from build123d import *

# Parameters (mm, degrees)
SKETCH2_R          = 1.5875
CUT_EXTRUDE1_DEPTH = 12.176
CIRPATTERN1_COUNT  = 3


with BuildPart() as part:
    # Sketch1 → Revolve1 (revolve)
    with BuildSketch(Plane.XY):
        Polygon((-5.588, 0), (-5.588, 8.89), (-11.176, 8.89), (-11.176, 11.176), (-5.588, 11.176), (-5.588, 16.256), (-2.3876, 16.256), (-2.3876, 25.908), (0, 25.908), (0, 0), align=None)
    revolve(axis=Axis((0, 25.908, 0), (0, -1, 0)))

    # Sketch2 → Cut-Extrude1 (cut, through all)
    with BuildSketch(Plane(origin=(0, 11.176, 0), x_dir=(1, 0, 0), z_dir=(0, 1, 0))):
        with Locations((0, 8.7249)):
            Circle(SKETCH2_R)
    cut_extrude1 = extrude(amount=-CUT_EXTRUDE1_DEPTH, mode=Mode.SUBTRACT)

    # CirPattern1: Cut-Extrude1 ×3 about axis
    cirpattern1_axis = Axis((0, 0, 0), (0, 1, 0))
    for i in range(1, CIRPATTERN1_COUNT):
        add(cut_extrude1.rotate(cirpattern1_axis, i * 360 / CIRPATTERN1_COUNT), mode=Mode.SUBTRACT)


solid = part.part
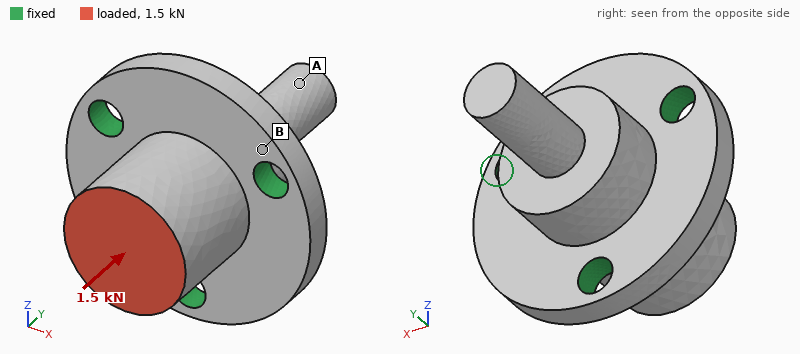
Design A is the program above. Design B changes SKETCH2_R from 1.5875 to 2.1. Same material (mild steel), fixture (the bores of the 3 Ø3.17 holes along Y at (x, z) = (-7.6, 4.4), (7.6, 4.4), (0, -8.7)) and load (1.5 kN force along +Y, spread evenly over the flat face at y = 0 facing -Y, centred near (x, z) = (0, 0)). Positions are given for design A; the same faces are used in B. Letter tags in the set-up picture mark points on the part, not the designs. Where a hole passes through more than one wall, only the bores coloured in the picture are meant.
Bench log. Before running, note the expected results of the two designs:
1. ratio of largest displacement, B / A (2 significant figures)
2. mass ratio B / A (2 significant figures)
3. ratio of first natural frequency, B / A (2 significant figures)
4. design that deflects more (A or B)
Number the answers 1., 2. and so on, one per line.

1. 0.77
2. 0.98
3. 1.1
4. A
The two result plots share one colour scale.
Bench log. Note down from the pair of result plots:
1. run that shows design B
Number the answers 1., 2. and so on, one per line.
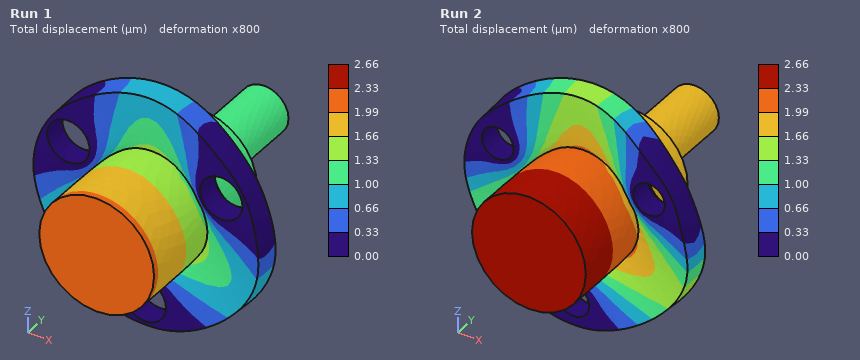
1. Run 1
